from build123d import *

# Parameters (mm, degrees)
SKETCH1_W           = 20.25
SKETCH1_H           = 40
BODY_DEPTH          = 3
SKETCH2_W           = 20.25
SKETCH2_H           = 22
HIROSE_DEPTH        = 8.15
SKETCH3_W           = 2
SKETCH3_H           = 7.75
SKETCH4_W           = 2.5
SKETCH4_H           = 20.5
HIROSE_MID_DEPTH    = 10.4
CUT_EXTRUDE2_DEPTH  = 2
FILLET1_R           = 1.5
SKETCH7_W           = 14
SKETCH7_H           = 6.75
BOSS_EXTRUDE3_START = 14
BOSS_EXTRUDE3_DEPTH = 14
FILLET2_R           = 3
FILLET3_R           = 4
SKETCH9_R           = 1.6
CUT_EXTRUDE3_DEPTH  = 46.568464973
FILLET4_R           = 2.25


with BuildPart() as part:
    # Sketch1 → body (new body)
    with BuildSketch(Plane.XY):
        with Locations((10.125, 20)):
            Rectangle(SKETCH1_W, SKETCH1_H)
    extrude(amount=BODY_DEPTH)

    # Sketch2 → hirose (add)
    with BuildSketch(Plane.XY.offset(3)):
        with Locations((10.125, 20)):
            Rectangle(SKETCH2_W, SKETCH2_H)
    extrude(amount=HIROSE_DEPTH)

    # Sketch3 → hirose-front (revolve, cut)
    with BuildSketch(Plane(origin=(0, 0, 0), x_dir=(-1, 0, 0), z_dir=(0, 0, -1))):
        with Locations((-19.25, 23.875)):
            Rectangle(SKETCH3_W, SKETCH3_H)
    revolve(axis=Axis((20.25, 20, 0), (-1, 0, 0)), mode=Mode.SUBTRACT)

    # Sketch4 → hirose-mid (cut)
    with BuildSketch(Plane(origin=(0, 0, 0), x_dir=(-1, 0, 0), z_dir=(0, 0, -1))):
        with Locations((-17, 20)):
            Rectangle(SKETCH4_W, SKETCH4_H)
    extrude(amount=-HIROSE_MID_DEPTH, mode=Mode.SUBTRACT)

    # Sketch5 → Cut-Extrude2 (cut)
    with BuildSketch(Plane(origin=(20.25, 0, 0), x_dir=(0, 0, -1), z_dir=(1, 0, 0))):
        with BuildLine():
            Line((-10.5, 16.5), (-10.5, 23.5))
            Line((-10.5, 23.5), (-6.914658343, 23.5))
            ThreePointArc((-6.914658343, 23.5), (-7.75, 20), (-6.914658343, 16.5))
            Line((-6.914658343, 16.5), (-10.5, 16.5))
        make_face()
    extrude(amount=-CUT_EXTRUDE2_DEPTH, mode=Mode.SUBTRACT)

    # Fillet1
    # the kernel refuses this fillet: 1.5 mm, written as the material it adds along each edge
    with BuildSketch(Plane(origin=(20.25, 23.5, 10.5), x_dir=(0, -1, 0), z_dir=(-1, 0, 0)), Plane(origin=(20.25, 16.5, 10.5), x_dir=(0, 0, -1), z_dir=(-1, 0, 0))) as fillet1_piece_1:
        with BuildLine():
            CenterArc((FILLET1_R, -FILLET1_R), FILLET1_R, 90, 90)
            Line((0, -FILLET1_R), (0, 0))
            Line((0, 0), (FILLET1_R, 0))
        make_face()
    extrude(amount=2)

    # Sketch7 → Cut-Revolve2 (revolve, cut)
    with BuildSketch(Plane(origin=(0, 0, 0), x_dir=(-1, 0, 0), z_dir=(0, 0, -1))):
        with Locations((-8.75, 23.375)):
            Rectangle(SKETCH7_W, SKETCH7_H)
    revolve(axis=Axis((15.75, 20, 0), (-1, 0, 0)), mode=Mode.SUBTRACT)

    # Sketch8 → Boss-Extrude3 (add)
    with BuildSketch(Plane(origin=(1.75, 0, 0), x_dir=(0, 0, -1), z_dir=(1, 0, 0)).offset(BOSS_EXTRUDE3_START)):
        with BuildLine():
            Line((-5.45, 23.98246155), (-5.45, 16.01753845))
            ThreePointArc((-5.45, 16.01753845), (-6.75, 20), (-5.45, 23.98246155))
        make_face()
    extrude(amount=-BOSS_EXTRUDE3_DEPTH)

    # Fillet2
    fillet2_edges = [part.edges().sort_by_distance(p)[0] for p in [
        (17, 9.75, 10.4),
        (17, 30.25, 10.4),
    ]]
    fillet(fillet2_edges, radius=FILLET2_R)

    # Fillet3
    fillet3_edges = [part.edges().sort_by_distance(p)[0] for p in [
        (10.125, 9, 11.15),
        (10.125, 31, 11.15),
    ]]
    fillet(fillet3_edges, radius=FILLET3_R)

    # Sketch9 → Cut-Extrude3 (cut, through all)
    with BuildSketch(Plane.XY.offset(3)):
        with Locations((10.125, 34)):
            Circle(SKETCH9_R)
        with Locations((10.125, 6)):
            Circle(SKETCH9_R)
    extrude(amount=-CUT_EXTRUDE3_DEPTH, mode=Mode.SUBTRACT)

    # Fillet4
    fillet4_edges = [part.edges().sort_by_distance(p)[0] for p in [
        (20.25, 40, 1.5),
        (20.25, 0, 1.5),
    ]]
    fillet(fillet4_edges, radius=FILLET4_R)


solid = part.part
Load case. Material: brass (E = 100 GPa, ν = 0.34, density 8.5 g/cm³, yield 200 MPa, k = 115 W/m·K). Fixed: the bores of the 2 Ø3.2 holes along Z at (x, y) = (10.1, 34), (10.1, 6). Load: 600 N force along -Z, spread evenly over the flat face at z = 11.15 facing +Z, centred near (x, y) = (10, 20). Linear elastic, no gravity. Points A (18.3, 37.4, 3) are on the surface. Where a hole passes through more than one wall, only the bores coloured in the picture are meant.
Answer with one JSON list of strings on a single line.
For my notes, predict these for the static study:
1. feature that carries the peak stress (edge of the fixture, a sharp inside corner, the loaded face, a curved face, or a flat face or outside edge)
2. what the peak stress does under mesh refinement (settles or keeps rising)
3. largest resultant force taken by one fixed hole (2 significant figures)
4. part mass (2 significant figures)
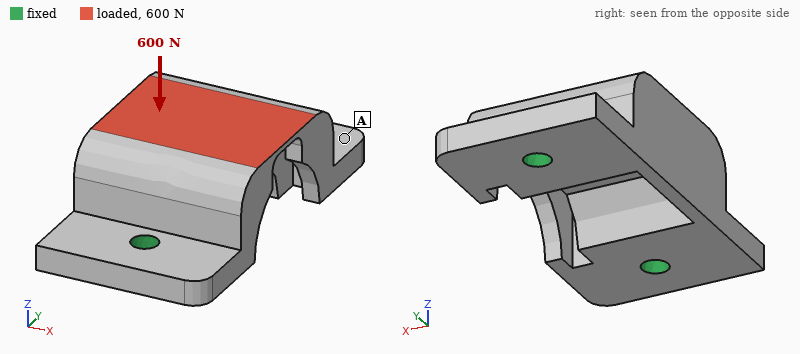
["edge of the fixture", "keeps rising", "400 N", "36 g"]
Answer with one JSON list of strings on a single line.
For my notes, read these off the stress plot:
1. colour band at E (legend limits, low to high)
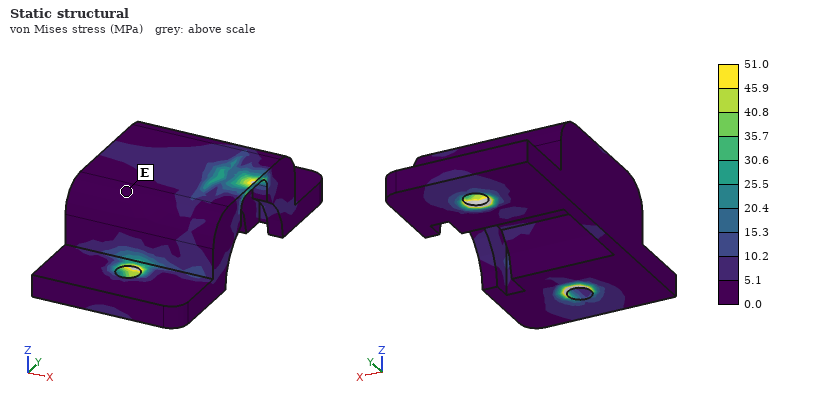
["0.0 to 5.1 MPa"]
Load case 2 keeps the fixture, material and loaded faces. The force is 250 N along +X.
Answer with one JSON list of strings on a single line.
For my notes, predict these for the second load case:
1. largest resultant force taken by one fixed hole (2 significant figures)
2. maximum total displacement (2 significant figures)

["130 N", "12 µm"]
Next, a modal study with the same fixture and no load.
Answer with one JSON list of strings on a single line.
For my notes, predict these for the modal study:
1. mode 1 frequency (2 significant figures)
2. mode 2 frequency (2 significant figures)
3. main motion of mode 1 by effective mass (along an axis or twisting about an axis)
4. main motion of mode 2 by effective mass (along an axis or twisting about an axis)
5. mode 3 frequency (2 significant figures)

["6400 Hz", "16 kHz", "along X", "along Z", "17 kHz"]
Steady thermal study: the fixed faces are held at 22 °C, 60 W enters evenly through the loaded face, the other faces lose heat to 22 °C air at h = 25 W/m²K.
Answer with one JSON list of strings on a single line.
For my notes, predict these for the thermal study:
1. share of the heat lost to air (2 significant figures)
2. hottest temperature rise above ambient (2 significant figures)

["3.2 %", "69 K"]
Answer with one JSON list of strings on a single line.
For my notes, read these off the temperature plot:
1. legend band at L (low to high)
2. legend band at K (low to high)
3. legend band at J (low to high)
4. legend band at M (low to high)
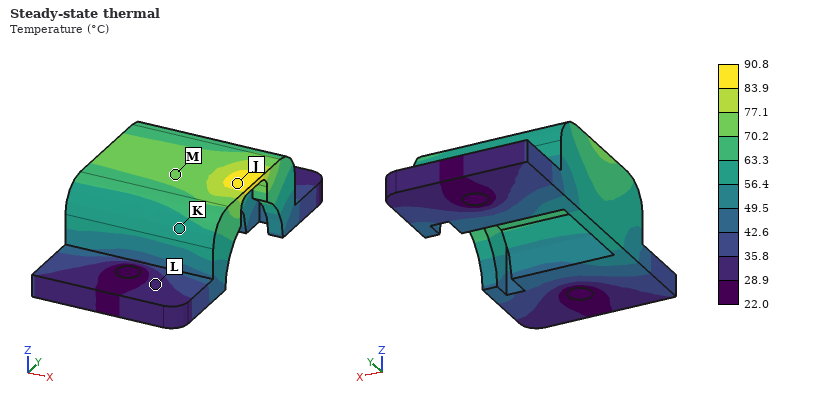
["28.9 to 35.8 °C", "56.4 to 63.3 °C", "83.9 to 90.8 °C", "70.2 to 77.1 °C"]
